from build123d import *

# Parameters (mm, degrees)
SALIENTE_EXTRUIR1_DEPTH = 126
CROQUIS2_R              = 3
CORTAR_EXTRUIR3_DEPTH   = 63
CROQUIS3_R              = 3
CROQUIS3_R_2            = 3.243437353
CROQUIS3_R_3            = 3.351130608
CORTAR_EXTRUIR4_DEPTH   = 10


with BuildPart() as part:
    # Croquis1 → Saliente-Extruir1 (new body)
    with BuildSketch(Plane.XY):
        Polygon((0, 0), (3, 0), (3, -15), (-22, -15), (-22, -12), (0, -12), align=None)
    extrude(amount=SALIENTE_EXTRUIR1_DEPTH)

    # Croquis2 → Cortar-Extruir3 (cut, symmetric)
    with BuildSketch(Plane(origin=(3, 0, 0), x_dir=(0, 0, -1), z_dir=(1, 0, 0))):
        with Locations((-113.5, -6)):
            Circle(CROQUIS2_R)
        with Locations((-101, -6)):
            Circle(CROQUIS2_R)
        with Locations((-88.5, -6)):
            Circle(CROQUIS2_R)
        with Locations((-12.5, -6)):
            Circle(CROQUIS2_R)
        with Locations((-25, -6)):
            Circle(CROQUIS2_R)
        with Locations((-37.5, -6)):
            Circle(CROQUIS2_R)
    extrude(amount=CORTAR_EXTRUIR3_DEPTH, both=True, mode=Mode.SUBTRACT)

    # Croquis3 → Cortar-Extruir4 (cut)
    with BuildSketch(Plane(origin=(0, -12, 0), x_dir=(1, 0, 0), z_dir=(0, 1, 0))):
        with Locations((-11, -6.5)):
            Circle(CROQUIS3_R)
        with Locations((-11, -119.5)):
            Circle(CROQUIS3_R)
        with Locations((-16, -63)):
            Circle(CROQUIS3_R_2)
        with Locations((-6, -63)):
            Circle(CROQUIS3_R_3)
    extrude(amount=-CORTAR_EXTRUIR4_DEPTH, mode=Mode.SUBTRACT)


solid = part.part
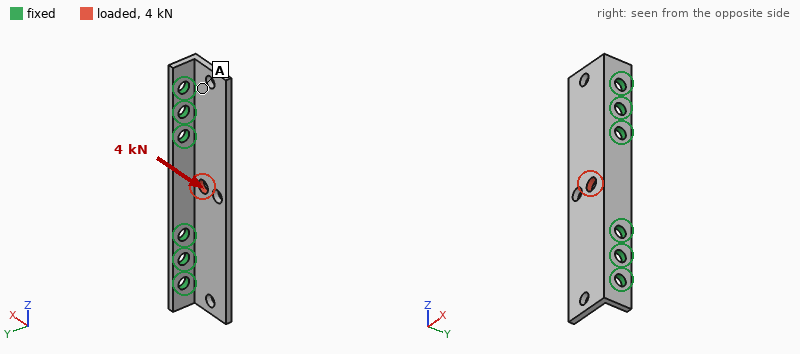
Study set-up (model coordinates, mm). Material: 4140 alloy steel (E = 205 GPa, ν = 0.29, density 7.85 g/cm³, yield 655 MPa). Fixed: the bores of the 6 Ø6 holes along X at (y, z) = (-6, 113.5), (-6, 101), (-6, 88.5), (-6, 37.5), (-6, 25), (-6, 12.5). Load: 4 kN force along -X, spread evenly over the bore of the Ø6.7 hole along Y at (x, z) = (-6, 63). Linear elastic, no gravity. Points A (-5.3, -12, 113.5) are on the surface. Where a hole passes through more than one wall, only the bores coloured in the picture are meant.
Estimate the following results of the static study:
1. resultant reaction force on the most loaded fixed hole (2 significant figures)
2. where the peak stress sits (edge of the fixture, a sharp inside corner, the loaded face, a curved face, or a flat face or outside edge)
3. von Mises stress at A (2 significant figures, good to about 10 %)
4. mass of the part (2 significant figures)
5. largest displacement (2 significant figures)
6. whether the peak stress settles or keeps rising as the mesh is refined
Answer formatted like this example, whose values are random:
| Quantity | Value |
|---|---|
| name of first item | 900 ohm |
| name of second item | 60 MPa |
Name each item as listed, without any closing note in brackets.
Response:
| Quantity | Value |
|---|---|
| resultant reaction force on the most loaded fixed hole | 1.8 kN |
| where the peak stress sits | edge of the fixture |
| von Mises stress at A | 28 MPa |
| mass of the part | 100 g |
| largest displacement | 68 µm |
| whether the peak stress settles or keeps rising as the mesh is refined | keeps rising |
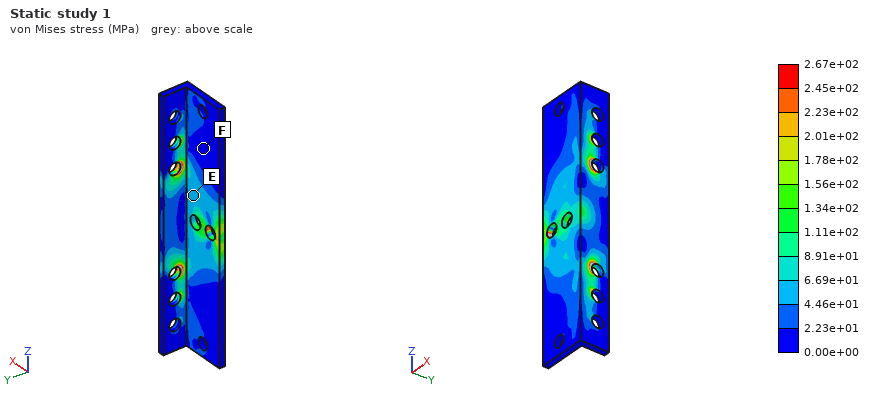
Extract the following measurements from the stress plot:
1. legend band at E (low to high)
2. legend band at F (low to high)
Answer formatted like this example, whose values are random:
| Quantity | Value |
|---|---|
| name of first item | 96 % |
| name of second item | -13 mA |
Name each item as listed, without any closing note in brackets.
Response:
| Quantity | Value |
|---|---|
| legend band at E | 4.46e+01 to 6.69e+01 MPa |
| legend band at F | 0.00e+00 to 2.23e+01 MPa |
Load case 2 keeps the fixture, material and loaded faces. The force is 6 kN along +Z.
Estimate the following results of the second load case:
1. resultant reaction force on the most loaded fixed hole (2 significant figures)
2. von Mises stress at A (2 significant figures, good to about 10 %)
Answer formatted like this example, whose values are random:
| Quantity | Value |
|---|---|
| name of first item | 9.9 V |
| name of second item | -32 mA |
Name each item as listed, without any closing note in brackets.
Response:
| Quantity | Value |
|---|---|
| resultant reaction force on the most loaded fixed hole | 2.1 kN |
| von Mises stress at A | 15 MPa |
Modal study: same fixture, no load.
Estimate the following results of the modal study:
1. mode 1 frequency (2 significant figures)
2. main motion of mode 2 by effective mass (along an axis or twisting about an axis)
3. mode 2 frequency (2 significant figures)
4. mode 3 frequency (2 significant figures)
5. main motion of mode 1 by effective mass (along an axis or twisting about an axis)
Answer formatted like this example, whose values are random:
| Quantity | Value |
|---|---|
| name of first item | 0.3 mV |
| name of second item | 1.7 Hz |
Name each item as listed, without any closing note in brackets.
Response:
| Quantity | Value |
|---|---|
| mode 1 frequency | 3100 Hz |
| main motion of mode 2 by effective mass | twisting about X |
| mode 2 frequency | 3800 Hz |
| mode 3 frequency | 4900 Hz |
| main motion of mode 1 by effective mass | along Y |
